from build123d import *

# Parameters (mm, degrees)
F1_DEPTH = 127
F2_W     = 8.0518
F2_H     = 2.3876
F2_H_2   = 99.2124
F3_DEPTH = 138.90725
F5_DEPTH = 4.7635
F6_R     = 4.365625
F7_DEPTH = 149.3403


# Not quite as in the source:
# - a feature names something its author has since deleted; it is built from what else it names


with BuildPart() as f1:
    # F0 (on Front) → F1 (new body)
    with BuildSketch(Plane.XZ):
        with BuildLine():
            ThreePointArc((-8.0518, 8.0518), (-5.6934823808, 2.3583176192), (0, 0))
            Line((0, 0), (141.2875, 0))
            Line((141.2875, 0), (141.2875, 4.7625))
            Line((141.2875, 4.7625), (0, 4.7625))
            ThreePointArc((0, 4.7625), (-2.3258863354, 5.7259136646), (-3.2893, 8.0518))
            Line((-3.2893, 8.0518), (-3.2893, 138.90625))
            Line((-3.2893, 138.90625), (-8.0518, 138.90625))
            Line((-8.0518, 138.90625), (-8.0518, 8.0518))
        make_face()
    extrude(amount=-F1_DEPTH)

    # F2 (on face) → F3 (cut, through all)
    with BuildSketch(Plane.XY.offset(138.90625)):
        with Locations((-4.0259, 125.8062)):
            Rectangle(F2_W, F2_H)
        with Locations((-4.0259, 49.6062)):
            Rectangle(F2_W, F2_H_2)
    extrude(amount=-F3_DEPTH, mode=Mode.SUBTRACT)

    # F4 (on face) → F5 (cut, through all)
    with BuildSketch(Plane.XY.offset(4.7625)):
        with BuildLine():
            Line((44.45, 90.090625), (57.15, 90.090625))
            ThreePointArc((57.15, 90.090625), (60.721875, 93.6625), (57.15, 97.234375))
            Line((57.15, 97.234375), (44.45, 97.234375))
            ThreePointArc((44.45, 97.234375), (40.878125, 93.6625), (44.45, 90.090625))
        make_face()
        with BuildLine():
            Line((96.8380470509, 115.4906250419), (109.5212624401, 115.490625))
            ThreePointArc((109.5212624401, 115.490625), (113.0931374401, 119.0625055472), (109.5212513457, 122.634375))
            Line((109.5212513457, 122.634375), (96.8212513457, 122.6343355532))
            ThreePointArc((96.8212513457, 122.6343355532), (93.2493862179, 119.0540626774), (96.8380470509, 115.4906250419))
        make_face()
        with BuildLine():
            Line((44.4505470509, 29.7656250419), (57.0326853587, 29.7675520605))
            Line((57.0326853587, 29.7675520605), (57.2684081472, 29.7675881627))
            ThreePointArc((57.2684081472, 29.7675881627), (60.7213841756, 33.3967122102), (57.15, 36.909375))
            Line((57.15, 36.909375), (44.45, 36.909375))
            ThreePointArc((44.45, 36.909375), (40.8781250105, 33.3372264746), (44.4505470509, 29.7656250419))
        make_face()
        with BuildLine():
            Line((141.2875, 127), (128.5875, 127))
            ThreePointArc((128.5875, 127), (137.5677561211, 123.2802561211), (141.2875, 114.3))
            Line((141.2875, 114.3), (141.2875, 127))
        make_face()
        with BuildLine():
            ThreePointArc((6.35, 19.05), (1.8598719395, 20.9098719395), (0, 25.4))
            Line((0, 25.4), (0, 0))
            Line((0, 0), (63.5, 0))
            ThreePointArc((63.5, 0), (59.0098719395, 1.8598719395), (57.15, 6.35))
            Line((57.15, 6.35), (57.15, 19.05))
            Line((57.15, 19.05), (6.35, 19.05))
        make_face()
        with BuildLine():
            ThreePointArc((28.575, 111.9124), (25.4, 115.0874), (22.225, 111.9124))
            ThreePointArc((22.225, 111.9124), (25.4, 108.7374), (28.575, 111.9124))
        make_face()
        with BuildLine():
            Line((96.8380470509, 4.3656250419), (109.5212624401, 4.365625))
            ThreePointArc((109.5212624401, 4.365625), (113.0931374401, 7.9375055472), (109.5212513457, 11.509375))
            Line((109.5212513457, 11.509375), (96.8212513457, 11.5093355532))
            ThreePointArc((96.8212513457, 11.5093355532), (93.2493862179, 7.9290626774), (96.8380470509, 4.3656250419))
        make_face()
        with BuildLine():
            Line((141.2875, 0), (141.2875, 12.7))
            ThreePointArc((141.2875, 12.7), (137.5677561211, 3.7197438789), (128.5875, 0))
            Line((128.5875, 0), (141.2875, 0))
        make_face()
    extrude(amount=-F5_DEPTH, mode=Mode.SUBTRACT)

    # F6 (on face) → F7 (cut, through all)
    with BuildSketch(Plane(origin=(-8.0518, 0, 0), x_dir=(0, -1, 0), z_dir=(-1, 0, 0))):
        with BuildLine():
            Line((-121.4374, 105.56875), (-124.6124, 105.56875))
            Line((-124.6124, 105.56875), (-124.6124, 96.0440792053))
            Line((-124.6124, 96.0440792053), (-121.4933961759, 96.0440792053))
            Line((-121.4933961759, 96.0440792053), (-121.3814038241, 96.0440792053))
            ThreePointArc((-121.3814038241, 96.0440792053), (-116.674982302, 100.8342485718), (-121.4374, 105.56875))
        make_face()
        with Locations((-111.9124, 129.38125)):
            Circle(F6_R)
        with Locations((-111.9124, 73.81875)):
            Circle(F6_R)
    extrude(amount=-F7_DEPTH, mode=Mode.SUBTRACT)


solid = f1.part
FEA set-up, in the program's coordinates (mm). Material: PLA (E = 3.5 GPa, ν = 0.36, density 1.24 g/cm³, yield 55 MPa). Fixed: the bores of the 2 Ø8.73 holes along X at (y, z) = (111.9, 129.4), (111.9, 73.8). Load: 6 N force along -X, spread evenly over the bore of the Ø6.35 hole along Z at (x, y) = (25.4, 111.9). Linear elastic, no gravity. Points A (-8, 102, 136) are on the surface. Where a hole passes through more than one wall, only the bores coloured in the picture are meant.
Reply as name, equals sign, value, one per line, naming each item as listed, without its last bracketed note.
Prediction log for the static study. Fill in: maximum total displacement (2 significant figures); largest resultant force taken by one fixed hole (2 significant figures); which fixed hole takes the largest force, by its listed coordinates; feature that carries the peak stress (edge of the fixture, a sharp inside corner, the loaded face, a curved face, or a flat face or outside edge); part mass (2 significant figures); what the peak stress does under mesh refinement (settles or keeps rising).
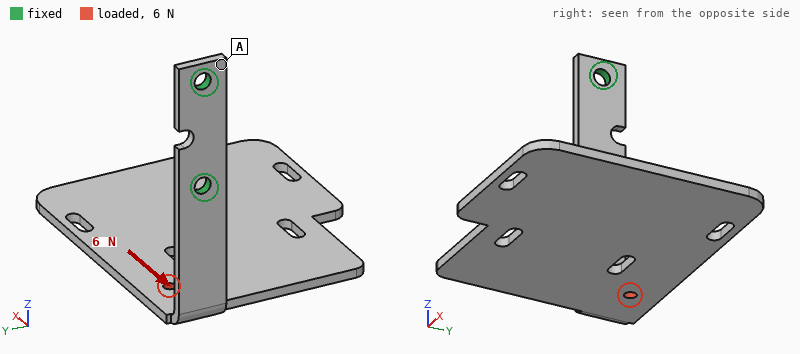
maximum total displacement = 2.7 mm
largest resultant force taken by one fixed hole = 5.9 N
which fixed hole takes the largest force, by its listed coordinates = (111.9, 73.8)
feature that carries the peak stress = edge of the fixture
part mass = 120 g
what the peak stress does under mesh refinement = keeps rising
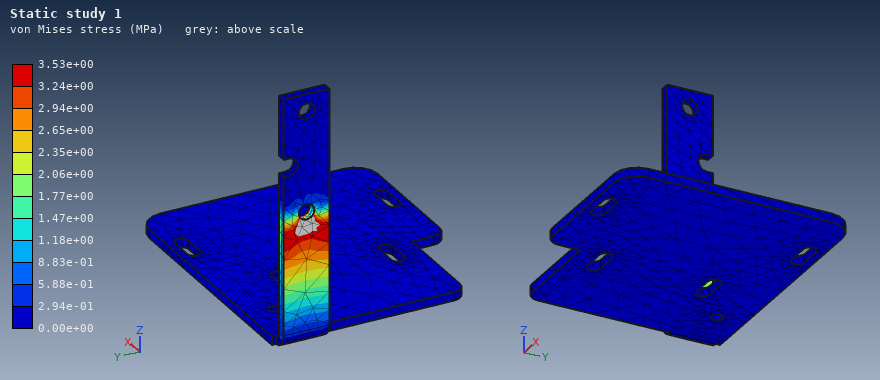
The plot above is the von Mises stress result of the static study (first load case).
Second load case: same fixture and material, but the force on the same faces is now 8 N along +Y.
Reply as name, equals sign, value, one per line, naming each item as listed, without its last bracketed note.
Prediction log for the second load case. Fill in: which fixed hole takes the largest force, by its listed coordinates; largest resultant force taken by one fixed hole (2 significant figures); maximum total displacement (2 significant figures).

which fixed hole takes the largest force, by its listed coordinates = (111.9, 73.8)
largest resultant force taken by one fixed hole = 13 N
maximum total displacement = 2.7 mm
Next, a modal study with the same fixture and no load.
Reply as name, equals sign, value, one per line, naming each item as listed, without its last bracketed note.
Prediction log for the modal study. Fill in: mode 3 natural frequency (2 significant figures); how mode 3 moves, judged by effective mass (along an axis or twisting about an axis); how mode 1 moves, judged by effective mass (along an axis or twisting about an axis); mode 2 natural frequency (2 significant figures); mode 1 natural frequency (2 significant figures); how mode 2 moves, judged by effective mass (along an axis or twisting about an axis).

mode 3 natural frequency = 68 Hz
how mode 3 moves, judged by effective mass = along X
how mode 1 moves, judged by effective mass = along Z
mode 2 natural frequency = 20 Hz
mode 1 natural frequency = 16 Hz
how mode 2 moves, judged by effective mass = along Y
